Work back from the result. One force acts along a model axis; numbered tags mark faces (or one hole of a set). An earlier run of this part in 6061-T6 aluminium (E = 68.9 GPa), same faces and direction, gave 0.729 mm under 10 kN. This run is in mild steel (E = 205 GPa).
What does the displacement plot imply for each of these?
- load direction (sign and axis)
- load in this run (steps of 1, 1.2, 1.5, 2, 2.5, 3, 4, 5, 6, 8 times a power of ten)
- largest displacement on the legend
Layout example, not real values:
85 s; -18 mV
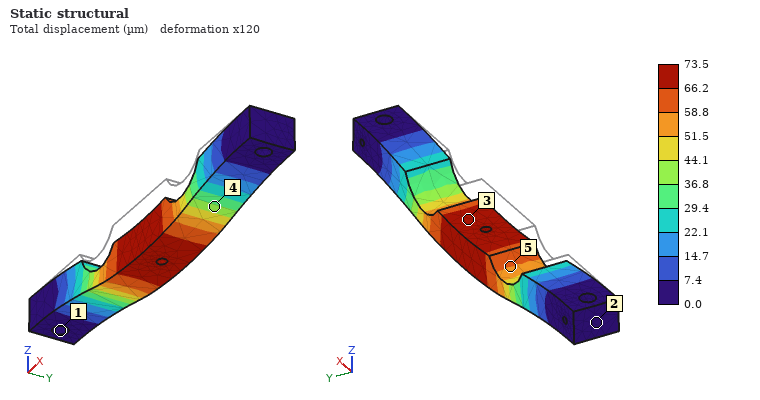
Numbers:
-Z; 3 kN; 73.5 µm
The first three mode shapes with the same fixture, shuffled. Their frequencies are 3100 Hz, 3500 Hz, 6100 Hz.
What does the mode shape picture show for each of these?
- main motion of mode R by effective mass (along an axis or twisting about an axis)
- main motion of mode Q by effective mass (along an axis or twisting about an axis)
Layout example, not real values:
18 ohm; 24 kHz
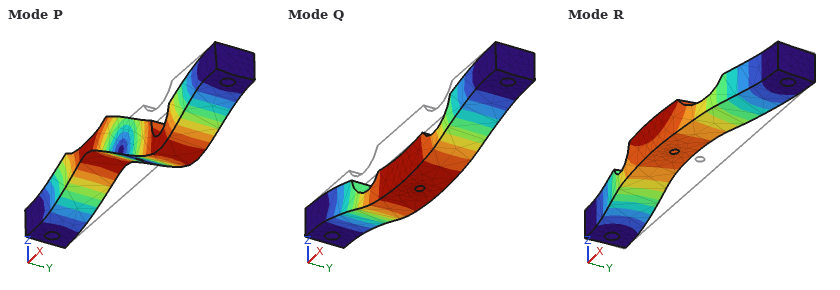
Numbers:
along Y; along Z
